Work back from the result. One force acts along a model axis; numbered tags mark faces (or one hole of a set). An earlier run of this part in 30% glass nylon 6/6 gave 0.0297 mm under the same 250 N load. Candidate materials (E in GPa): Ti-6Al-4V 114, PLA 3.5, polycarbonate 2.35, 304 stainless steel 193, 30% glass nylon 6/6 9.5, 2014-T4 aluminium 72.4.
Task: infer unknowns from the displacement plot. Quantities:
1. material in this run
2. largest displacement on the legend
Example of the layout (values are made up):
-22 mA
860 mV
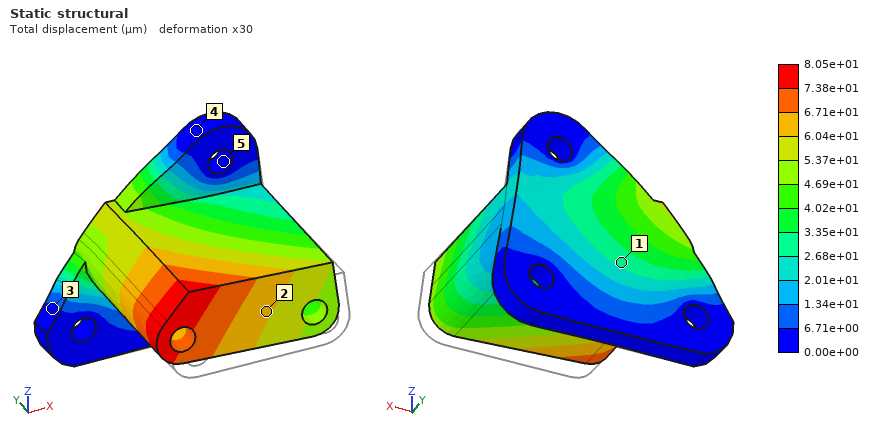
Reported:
PLA
8.05e+01 µm
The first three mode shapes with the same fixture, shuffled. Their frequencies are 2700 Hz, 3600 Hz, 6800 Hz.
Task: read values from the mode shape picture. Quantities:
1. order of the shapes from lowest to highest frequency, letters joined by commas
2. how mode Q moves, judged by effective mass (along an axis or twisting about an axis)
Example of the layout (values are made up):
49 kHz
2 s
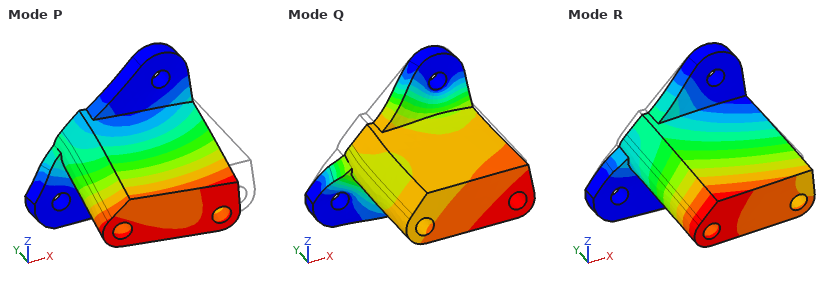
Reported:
R, P, Q
along Y
